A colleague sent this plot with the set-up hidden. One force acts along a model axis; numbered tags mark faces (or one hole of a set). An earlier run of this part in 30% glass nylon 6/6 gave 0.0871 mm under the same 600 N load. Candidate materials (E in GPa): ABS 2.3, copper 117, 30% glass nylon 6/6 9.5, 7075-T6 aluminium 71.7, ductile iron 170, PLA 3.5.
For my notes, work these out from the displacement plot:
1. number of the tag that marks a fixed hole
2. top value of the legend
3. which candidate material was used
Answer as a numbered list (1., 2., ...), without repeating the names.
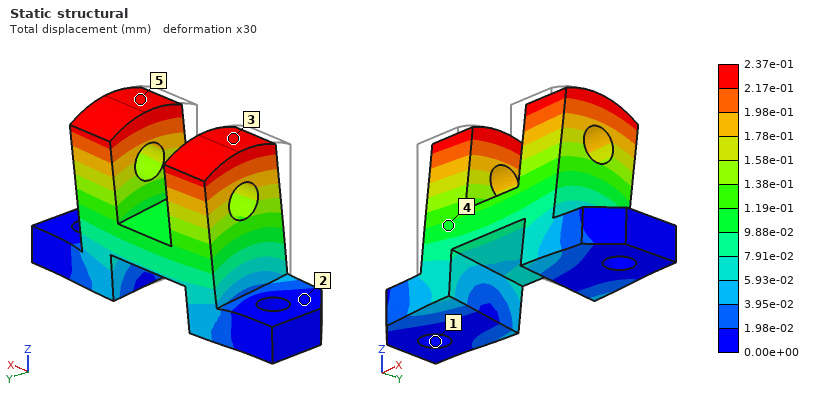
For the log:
1. 1
2. 2.37e-01 mm
3. PLA
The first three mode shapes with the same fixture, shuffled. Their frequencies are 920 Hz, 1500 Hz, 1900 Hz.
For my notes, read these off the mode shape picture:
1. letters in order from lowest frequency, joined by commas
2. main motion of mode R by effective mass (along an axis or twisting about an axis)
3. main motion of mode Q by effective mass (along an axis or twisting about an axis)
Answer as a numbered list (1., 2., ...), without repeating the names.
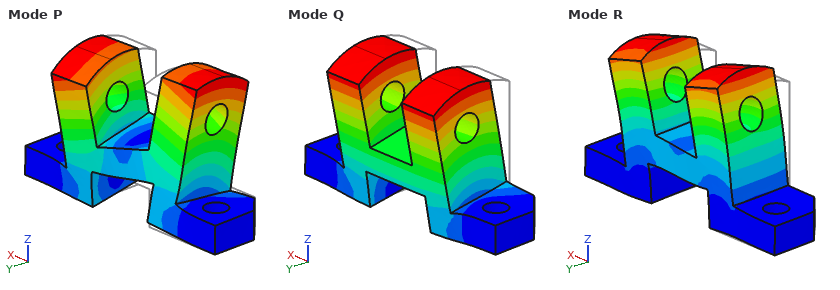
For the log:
1. Q, P, R
2. along X
3. along Y
